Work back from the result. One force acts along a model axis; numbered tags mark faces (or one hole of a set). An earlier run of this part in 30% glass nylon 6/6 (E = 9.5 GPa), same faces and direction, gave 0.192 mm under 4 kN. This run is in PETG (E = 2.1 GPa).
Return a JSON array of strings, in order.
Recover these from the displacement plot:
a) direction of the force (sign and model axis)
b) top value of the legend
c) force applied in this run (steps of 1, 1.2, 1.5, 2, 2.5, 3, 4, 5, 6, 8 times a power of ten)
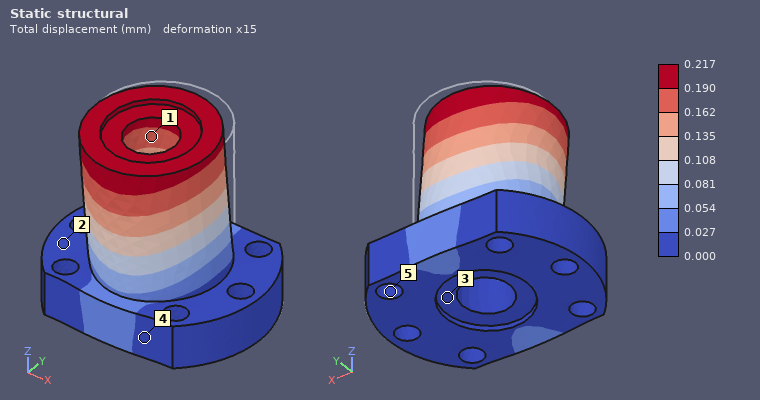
["-Y", "0.217 mm", "1 kN"]
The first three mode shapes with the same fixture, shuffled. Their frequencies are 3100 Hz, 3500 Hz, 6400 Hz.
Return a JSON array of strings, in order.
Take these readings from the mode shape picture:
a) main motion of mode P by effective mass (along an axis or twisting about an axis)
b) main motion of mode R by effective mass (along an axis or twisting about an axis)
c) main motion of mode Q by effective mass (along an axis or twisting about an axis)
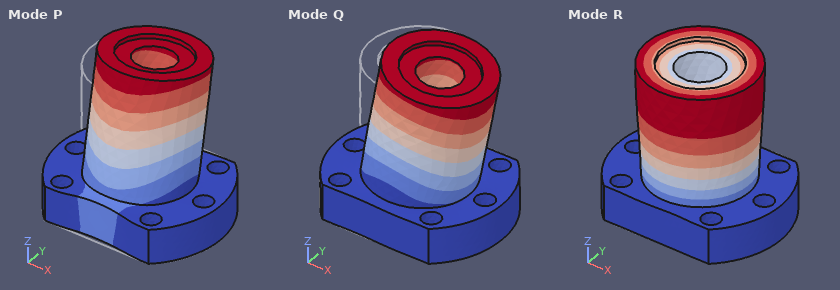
["along Y", "twisting about Z", "along X"]
